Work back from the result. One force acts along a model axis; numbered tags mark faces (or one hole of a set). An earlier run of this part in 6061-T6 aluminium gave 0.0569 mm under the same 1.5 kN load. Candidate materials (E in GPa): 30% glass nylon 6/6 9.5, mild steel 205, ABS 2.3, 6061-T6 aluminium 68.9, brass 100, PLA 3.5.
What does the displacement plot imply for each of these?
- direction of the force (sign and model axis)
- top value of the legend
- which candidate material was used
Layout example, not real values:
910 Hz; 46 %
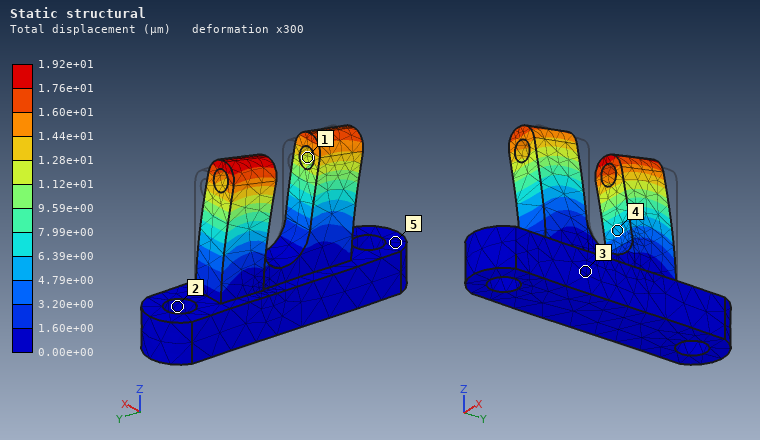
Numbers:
-Y; 1.92e+01 µm; mild steel
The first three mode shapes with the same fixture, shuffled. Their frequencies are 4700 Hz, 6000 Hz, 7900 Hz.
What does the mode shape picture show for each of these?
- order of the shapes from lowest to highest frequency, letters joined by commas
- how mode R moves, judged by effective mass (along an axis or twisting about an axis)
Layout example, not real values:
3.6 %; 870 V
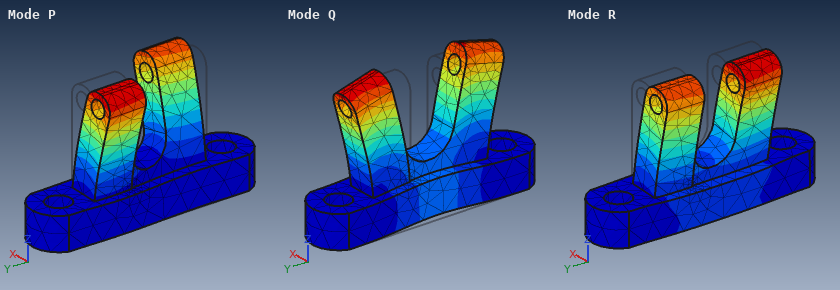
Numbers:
R, P, Q; along X
